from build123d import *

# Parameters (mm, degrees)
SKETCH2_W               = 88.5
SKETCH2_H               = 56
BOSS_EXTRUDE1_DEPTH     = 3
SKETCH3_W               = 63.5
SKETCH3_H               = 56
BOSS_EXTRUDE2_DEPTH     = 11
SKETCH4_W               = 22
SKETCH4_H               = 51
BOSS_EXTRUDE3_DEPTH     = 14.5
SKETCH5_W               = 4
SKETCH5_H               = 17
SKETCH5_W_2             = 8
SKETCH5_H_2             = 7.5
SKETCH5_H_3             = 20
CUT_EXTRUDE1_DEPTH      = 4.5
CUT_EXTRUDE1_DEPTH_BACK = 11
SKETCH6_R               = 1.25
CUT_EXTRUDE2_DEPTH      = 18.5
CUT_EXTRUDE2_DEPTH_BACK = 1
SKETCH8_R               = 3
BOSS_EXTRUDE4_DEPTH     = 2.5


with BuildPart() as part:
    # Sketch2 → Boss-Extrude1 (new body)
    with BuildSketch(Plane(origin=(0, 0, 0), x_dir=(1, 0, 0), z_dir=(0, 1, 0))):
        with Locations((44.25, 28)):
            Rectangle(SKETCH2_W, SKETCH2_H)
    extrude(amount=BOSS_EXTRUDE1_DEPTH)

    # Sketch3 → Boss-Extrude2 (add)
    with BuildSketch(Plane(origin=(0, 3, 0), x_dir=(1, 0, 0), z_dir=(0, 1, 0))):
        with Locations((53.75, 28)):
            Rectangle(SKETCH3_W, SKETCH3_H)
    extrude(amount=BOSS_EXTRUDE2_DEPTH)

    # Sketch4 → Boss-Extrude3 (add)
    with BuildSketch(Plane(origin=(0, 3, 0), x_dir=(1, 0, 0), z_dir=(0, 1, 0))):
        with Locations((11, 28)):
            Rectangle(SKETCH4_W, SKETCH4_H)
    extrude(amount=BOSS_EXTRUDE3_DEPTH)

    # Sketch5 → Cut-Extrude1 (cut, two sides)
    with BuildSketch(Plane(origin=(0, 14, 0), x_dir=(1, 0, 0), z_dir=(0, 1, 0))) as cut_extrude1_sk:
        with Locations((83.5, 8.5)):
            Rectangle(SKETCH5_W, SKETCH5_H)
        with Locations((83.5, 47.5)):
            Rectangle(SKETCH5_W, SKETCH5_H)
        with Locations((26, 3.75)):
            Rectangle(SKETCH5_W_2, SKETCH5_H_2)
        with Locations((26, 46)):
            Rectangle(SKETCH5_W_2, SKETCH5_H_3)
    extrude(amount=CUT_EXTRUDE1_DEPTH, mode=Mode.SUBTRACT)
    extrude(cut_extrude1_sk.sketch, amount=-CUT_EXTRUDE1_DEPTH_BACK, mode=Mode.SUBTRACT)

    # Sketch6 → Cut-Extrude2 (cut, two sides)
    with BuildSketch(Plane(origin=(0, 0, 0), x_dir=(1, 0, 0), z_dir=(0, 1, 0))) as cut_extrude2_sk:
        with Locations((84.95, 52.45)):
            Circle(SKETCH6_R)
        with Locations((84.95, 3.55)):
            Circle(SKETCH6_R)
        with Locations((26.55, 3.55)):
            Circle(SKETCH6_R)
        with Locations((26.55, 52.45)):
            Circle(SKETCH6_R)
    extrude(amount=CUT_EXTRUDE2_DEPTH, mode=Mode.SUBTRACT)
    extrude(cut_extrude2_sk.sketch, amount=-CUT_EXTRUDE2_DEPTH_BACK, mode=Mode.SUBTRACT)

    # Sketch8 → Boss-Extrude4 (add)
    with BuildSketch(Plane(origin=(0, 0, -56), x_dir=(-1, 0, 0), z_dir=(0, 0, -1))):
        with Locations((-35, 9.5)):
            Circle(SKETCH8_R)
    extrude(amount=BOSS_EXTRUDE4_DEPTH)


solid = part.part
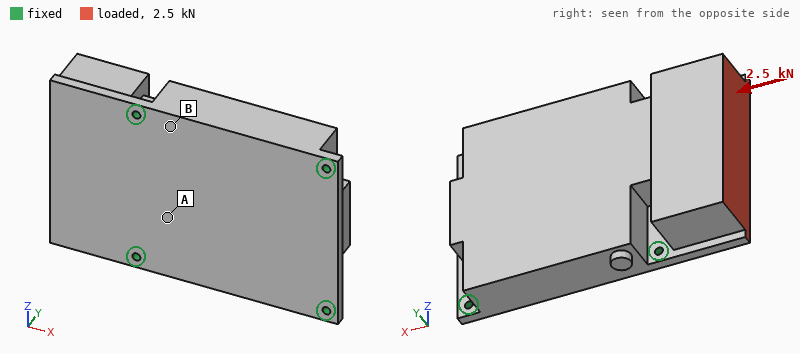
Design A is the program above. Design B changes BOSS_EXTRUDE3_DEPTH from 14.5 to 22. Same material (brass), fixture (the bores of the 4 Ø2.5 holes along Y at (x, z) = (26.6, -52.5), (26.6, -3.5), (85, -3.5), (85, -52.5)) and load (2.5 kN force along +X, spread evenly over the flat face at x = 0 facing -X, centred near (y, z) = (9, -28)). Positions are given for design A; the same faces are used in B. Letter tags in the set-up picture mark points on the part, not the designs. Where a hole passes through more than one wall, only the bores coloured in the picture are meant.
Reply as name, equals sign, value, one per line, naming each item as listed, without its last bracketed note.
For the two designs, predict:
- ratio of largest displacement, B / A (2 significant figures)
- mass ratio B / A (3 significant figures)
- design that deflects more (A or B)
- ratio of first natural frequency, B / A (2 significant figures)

ratio of largest displacement, B / A = 1.7
mass ratio B / A = 1.13
design that deflects more = B
ratio of first natural frequency, B / A = 0.81
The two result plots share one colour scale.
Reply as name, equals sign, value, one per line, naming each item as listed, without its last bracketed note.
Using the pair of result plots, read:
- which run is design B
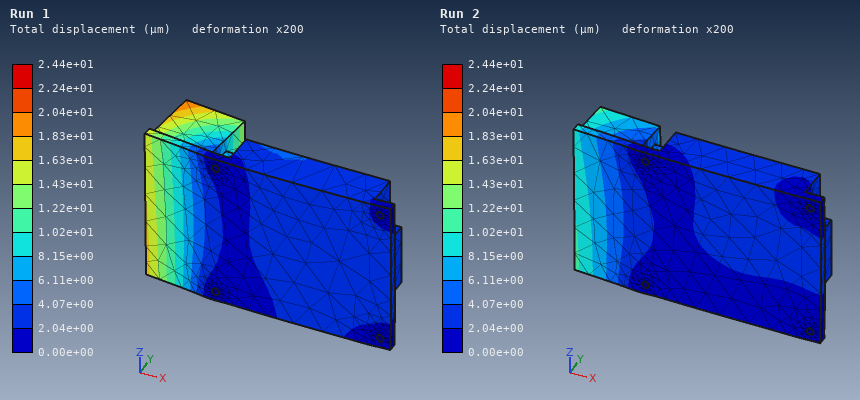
which run is design B = Run 1
